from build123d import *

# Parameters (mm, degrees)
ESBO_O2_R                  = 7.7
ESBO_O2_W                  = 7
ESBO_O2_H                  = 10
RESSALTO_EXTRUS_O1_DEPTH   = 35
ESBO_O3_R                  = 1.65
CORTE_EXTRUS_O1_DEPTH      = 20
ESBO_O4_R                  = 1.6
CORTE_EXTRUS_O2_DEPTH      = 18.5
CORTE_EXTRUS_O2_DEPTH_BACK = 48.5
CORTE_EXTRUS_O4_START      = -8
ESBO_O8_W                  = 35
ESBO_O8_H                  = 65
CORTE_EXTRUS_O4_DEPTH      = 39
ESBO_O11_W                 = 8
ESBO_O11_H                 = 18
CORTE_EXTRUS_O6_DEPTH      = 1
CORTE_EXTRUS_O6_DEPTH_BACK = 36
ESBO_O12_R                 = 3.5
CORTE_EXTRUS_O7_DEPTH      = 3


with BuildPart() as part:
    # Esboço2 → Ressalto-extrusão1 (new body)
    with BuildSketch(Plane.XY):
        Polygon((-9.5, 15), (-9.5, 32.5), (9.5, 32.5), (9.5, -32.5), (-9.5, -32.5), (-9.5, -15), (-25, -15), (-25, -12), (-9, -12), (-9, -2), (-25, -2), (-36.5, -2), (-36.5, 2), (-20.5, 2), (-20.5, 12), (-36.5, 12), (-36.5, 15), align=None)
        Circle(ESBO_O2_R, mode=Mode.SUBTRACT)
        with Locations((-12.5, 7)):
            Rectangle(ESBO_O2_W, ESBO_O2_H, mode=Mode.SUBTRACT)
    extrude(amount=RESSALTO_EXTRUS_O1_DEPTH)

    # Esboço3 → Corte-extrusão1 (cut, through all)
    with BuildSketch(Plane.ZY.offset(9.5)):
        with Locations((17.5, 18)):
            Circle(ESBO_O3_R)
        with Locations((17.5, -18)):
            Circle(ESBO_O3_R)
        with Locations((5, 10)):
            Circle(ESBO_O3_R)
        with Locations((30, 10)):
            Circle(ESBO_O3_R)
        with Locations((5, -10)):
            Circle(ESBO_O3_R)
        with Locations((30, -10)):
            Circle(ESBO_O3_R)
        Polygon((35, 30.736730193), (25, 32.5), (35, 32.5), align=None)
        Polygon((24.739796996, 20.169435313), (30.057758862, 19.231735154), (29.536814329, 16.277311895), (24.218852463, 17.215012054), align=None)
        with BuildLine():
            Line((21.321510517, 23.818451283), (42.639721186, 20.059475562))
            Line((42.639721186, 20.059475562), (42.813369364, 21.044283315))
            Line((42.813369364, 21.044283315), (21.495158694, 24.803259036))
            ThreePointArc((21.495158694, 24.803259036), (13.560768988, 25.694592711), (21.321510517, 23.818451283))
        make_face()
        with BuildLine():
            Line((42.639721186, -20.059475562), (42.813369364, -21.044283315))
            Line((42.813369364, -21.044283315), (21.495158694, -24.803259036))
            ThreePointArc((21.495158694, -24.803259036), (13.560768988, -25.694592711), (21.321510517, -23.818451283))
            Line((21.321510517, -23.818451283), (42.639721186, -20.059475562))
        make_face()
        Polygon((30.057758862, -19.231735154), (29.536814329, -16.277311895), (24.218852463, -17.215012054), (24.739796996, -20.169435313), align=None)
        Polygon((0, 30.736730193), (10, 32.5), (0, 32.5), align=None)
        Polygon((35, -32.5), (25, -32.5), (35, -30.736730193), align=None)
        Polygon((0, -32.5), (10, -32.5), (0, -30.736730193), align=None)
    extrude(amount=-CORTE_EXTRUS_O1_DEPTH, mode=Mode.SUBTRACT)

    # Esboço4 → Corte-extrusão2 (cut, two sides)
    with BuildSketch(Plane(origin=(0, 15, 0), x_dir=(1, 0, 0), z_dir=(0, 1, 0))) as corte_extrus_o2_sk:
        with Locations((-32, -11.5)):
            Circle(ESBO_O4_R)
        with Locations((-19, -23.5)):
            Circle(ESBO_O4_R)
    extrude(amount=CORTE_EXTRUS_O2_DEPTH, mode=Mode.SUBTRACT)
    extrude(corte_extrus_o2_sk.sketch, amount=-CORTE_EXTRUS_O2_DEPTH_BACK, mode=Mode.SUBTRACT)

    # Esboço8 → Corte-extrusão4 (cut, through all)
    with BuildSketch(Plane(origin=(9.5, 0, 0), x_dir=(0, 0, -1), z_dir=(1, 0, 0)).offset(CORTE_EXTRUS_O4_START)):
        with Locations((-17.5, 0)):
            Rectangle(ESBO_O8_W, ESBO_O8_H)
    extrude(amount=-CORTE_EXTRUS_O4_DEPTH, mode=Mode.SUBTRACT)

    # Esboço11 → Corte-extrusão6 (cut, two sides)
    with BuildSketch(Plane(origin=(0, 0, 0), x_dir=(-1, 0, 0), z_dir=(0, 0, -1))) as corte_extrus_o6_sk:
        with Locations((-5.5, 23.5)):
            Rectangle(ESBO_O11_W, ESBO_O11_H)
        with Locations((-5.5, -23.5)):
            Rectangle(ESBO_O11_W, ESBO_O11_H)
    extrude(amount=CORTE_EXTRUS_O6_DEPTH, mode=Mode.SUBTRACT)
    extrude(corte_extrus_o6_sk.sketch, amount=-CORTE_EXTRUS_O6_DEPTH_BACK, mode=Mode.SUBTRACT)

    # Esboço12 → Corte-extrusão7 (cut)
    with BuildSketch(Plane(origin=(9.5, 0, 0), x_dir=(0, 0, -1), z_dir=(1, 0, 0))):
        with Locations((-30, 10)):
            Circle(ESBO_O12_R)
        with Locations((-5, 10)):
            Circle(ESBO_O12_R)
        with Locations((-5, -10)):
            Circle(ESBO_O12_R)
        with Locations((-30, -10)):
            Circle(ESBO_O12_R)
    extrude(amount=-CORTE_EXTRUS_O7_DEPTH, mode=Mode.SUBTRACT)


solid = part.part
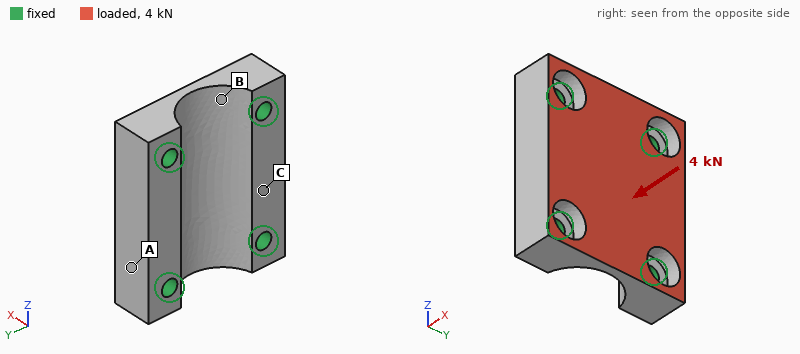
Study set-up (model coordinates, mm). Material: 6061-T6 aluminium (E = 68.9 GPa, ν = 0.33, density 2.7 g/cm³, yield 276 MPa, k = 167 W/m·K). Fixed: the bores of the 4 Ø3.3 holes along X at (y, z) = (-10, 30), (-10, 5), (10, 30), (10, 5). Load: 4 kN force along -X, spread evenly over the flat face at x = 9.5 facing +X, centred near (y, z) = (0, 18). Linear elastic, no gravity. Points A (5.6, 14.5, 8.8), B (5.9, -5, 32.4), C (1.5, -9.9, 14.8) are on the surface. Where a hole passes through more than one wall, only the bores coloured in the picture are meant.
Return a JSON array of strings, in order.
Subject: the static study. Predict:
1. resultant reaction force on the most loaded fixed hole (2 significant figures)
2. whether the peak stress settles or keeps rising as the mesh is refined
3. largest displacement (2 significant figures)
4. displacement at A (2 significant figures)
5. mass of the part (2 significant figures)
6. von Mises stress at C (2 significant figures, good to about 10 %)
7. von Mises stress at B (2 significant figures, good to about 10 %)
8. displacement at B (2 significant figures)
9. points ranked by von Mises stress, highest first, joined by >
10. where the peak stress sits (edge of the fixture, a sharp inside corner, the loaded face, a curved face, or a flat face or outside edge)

["1.2 kN", "keeps rising", "13 µm", "2.0 µm", "14 g", "17 MPa", "27 MPa", "2.7 µm", "B > C > A", "edge of the fixture"]
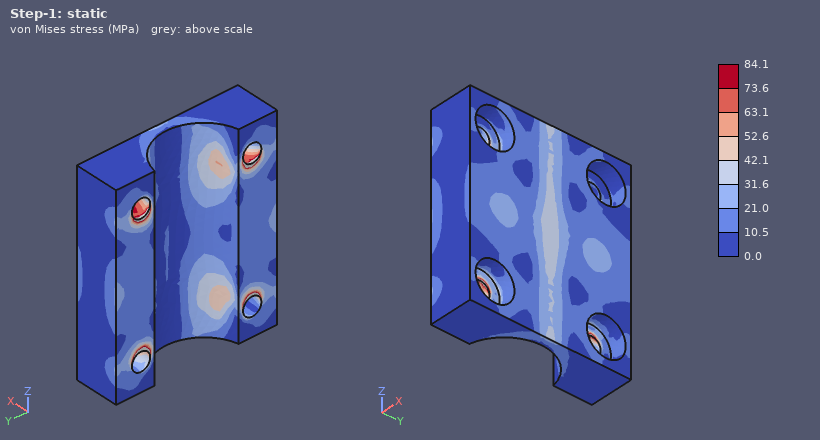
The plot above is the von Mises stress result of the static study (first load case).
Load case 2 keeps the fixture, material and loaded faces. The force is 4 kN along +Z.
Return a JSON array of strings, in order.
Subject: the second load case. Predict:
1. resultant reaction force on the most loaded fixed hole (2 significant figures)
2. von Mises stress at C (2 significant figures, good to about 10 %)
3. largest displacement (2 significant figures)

["1.1 kN", "6.5 MPa", "8.4 µm"]
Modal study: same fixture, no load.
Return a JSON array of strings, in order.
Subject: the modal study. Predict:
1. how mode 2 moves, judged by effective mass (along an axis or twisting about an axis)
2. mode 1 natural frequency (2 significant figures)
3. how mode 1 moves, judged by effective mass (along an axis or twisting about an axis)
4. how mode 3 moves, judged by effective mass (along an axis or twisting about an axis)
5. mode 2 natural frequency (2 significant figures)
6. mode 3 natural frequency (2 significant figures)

["along Y", "36 kHz", "along X", "along Y", "38 kHz", "41 kHz"]
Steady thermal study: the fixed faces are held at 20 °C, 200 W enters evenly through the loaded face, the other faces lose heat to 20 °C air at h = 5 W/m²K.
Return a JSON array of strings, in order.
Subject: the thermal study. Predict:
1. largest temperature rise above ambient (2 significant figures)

["41 K"]
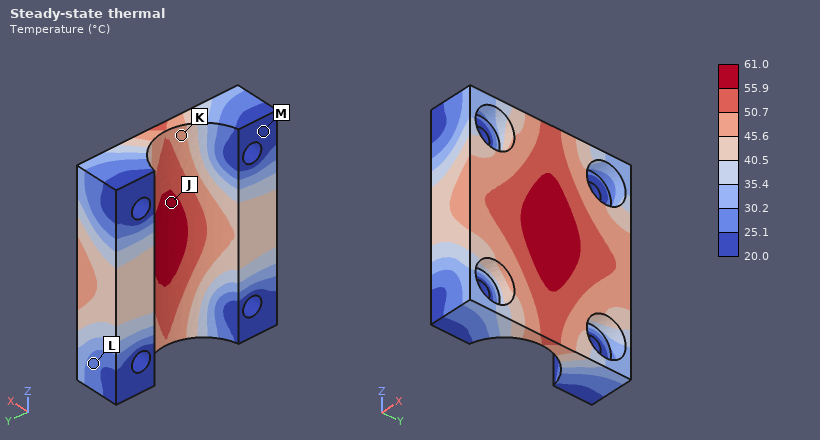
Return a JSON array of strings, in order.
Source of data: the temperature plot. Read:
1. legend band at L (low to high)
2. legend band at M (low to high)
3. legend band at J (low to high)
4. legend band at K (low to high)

["25.1 to 30.2 °C", "20.0 to 25.1 °C", "55.9 to 61.0 °C", "45.6 to 50.7 °C"]
